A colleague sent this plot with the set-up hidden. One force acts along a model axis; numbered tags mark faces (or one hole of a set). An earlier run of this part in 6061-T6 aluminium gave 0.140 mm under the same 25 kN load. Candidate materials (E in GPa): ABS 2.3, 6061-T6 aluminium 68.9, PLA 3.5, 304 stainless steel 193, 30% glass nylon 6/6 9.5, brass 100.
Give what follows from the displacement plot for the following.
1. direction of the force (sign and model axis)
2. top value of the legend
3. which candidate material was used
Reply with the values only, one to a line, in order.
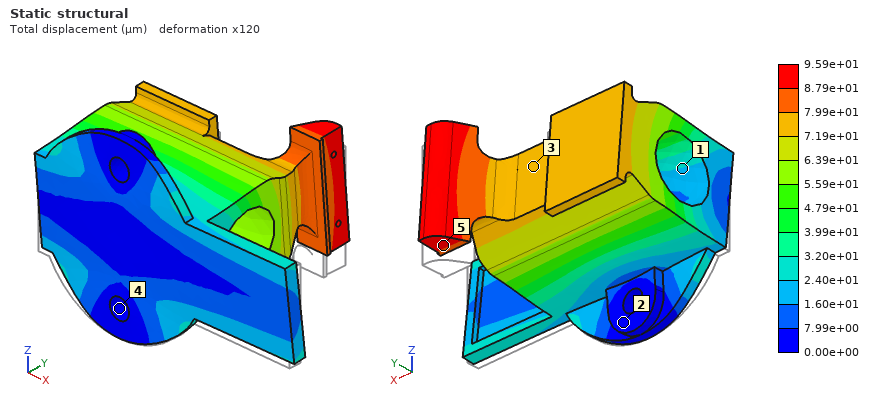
+Z
9.59e+01 µm
brass
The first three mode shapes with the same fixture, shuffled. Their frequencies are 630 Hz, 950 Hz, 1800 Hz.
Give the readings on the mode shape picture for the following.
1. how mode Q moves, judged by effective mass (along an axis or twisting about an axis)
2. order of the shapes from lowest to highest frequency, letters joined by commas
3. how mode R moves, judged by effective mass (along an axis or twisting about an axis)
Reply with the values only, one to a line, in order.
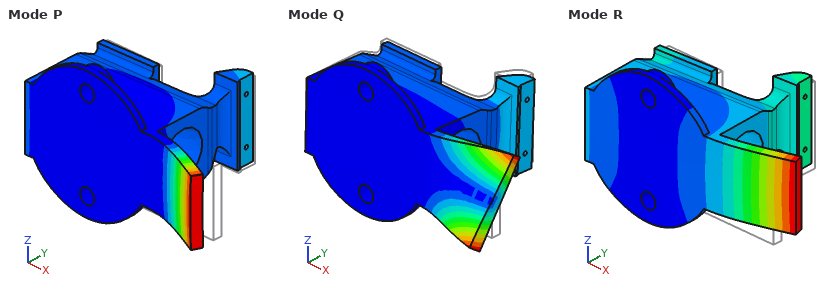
along Z
R, P, Q
along X
